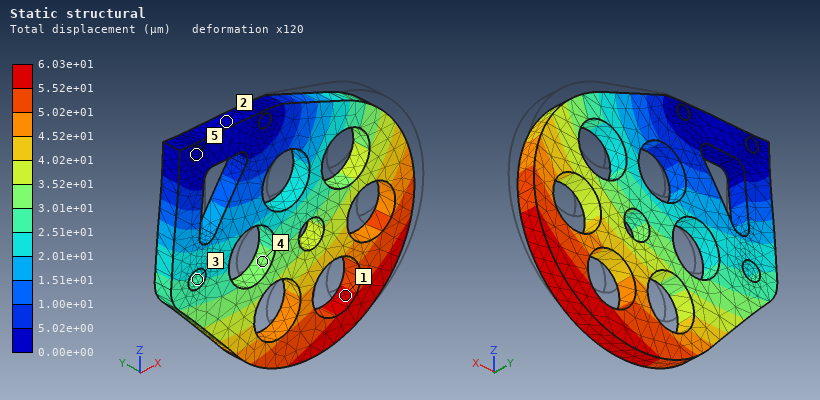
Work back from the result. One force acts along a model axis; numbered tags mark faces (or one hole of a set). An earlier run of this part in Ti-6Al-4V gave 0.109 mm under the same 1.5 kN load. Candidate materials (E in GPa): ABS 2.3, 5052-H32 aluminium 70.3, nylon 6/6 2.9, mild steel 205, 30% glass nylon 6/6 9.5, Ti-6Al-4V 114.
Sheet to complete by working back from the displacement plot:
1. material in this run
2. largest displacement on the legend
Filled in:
mild steel
6.03e+01 µm
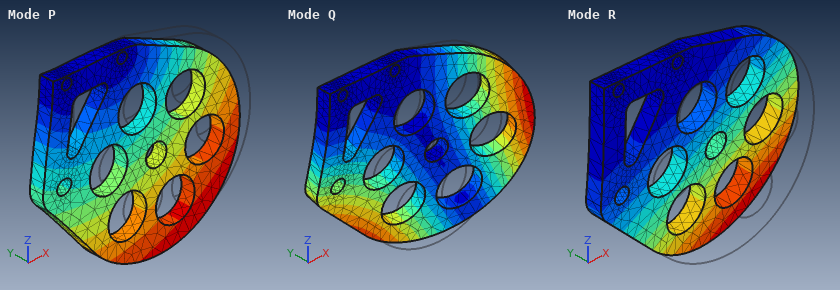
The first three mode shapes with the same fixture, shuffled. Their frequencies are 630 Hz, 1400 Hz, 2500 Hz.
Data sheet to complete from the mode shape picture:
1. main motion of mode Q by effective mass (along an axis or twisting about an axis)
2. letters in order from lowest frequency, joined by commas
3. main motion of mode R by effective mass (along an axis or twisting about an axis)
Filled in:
twisting about Z
R, Q, P
along Y
